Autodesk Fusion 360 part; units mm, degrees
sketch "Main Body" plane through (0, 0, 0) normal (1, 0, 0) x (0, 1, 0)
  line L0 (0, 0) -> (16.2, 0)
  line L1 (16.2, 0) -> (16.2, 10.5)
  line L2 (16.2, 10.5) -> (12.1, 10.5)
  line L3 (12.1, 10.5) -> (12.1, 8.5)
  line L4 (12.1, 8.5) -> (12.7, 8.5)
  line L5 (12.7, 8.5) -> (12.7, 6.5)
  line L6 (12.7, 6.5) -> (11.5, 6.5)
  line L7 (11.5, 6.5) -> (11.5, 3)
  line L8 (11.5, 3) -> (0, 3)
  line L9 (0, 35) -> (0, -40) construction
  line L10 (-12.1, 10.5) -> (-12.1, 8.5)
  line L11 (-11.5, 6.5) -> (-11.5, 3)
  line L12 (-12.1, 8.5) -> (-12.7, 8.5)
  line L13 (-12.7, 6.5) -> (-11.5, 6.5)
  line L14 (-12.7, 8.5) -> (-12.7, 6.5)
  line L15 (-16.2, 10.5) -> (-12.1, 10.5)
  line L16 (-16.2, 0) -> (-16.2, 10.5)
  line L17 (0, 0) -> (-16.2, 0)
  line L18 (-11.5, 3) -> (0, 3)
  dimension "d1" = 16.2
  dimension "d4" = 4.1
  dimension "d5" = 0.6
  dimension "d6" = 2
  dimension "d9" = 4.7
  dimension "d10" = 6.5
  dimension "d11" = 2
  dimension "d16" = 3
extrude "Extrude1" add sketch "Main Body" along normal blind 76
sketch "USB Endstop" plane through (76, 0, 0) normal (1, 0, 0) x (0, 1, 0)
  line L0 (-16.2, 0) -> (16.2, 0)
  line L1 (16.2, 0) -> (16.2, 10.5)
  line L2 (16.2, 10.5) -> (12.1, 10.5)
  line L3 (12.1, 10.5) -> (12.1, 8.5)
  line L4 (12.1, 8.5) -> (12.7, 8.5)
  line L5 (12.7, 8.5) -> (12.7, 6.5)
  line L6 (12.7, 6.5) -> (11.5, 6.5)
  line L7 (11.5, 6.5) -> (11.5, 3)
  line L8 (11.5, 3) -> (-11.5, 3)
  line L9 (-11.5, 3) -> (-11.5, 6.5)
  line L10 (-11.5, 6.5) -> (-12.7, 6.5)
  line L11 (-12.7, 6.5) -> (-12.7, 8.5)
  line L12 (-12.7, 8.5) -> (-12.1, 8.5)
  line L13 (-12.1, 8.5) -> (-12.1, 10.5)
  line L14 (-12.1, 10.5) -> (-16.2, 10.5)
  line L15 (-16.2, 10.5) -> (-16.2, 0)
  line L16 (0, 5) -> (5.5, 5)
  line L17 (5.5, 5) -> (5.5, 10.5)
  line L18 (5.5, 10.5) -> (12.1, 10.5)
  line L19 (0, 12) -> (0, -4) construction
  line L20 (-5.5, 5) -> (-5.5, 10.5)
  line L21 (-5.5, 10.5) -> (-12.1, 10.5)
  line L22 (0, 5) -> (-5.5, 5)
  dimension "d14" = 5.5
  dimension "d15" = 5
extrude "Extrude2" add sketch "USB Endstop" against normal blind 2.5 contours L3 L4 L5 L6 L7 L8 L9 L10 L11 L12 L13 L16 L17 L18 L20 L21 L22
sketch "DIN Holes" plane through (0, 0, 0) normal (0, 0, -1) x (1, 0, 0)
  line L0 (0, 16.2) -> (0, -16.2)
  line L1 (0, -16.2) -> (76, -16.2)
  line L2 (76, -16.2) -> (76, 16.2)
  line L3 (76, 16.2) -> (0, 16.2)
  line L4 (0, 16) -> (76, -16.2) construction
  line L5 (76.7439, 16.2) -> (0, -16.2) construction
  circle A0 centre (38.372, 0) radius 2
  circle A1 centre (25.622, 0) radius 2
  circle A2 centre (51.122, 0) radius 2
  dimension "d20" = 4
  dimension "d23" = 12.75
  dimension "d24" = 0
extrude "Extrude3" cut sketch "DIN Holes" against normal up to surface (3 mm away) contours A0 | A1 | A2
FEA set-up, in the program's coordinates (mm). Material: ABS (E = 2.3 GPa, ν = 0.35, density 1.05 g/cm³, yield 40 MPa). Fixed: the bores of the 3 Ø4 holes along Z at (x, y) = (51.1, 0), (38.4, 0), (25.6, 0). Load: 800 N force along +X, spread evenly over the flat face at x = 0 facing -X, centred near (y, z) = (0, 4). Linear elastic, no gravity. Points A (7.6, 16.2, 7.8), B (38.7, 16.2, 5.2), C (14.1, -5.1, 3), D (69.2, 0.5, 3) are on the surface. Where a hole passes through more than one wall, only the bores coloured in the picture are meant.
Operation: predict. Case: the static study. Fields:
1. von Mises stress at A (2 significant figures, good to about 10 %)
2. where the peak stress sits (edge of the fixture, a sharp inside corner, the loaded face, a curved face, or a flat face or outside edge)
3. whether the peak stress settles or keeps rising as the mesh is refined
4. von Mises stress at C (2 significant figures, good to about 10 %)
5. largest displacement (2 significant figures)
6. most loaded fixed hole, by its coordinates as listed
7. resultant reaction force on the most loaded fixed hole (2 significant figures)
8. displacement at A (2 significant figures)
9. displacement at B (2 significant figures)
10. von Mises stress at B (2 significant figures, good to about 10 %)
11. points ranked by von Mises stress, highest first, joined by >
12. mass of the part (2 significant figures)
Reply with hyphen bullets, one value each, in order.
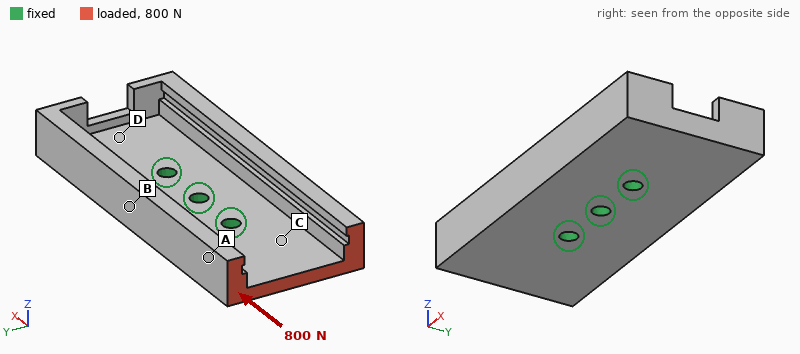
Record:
- 5.0 MPa
- edge of the fixture
- keeps rising
- 6.5 MPa
- 0.29 mm
- (25.6, 0)
- 440 N
- 0.22 mm
- 0.048 mm
- 2.5 MPa
- C > A > B > D
- 13 g
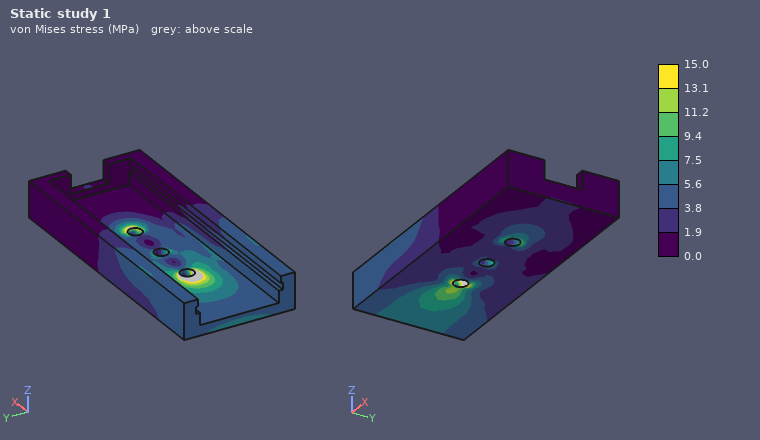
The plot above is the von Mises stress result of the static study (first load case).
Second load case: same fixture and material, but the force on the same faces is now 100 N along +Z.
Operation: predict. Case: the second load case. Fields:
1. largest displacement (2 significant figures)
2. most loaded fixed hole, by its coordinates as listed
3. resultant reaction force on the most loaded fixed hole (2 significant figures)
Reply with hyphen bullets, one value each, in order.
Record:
- 0.85 mm
- (25.6, 0)
- 180 N
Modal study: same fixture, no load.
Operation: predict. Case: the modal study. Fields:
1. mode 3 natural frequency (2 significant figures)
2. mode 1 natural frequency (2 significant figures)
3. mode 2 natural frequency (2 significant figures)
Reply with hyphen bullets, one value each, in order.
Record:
- 1200 Hz
- 1100 Hz
- 1200 Hz
